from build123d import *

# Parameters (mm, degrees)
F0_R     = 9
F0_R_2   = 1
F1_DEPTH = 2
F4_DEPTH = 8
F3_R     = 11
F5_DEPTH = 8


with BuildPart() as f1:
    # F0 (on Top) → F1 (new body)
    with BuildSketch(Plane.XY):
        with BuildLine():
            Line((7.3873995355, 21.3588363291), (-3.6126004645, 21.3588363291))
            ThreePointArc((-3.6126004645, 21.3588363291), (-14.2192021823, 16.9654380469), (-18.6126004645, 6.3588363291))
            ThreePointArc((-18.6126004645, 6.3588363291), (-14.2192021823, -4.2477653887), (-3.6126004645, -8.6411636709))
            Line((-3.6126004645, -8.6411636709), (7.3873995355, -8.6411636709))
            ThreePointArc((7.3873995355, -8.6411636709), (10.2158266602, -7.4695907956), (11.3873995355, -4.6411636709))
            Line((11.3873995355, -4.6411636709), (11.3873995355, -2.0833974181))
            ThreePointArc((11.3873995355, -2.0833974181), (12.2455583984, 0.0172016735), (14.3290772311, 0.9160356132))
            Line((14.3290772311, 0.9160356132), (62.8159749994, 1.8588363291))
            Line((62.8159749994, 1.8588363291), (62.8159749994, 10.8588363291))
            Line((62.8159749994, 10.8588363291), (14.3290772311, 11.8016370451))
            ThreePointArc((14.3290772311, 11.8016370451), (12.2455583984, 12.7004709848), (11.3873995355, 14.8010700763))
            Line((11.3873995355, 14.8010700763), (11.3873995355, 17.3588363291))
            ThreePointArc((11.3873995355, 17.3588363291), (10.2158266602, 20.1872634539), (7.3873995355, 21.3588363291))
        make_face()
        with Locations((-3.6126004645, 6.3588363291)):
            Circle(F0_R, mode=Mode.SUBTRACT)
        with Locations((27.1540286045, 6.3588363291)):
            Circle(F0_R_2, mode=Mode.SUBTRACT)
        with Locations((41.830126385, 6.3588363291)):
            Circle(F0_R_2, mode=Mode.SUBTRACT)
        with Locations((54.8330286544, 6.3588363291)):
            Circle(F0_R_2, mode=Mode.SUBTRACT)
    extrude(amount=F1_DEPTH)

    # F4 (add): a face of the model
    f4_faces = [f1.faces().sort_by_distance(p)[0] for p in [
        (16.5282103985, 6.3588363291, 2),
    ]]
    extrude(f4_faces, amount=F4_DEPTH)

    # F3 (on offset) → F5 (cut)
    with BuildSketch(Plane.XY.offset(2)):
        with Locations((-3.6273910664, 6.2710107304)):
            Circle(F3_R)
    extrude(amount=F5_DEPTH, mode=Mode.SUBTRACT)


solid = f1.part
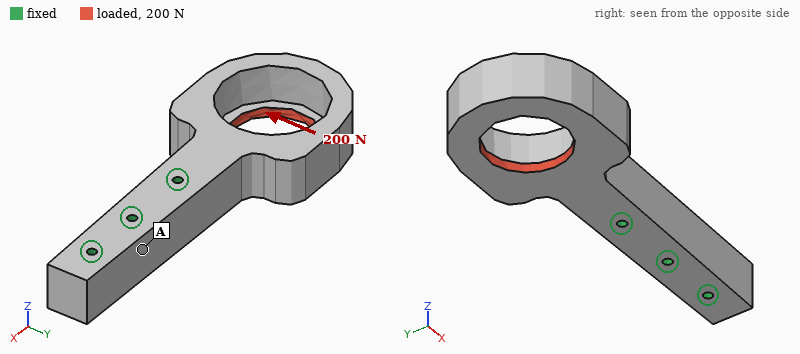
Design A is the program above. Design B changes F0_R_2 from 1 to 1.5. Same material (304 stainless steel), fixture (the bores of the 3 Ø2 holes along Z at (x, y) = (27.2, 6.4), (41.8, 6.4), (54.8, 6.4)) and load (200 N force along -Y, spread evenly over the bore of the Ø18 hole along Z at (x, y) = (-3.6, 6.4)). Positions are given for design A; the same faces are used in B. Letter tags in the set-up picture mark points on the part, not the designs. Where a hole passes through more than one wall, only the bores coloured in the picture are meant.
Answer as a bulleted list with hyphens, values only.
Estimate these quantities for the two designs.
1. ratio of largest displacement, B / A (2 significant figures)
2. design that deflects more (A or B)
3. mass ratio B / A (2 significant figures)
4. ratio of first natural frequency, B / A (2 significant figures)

- 0.91
- A
- 0.99
- 1.1
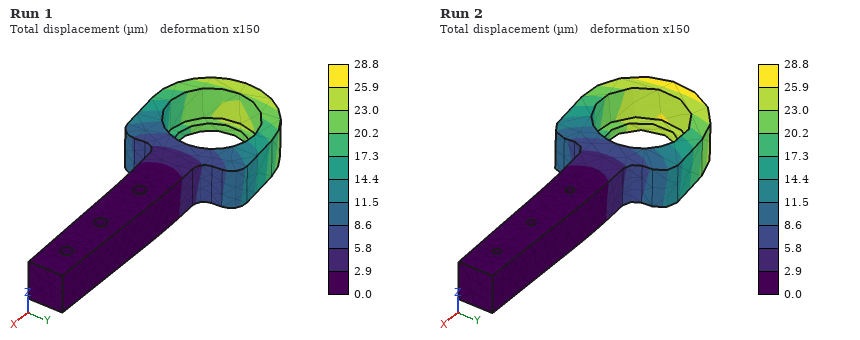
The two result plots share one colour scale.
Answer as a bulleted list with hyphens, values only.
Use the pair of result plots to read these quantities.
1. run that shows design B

- Run 1
